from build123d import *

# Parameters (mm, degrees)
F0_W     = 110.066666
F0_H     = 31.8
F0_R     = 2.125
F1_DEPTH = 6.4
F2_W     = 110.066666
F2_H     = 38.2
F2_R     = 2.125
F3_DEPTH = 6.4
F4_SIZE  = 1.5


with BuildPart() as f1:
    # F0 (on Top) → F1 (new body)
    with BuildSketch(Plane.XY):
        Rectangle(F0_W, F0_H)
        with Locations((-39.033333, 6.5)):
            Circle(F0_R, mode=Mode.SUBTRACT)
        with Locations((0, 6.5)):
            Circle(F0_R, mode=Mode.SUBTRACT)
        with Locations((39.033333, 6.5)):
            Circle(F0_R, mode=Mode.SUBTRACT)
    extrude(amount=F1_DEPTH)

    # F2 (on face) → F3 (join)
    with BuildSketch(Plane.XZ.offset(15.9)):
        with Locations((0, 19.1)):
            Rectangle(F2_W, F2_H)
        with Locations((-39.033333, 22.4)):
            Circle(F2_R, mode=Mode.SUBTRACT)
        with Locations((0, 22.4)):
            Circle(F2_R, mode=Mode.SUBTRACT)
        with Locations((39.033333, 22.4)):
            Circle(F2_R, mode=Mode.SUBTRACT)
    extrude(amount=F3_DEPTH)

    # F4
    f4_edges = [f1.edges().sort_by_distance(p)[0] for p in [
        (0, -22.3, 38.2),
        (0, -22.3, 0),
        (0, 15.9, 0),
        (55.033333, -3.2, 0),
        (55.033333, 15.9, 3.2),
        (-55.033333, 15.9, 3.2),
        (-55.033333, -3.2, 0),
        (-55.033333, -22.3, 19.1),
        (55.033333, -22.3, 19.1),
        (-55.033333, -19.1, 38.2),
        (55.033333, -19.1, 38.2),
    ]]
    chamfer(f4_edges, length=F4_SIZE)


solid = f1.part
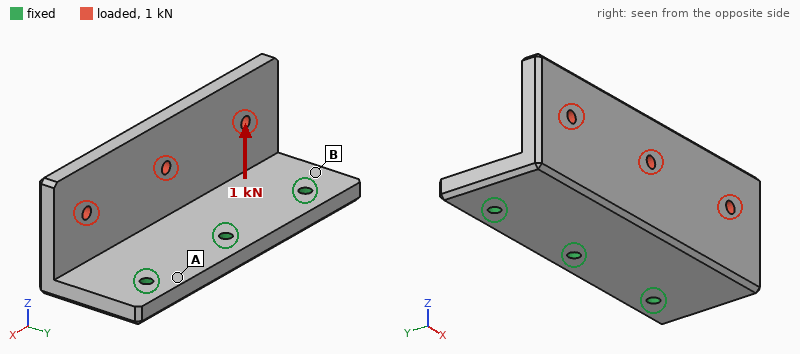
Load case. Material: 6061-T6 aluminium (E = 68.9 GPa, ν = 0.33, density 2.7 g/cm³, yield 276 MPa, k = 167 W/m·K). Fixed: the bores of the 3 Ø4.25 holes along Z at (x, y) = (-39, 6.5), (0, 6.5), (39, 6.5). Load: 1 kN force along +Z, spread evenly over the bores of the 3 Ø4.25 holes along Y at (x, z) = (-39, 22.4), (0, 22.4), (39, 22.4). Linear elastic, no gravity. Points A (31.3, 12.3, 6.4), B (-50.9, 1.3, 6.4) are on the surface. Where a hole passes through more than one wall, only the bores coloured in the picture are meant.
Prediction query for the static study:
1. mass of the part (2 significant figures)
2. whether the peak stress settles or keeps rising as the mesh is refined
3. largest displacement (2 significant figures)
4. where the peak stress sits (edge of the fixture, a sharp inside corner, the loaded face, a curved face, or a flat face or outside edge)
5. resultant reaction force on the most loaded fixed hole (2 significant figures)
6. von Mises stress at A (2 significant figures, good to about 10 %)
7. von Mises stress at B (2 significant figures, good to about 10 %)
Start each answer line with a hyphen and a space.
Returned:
- 130 g
- keeps rising
- 0.10 mm
- edge of the fixture
- 350 N
- 9.4 MPa
- 20 MPa
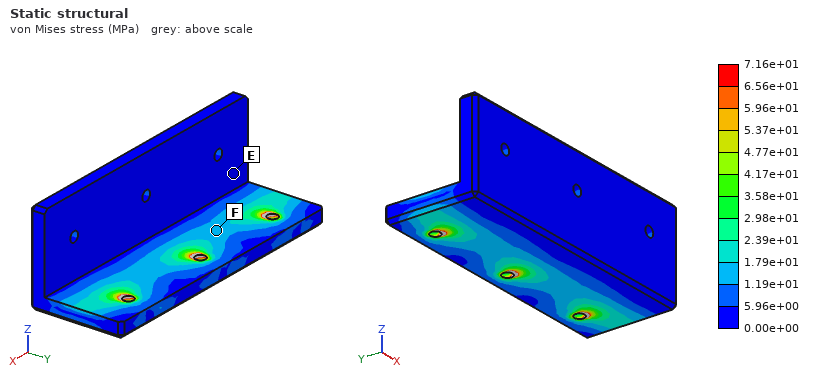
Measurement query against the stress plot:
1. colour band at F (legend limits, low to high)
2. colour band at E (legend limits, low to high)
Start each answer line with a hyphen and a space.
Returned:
- 1.19e+01 to 1.79e+01 MPa
- 0.00e+00 to 5.96e+00 MPa
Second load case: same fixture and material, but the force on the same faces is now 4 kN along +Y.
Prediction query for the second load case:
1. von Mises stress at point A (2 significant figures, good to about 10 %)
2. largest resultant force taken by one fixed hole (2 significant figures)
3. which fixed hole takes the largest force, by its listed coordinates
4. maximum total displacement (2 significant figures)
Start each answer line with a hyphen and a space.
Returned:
- 34 MPa
- 1.5 kN
- (0, 6.5)
- 0.58 mm
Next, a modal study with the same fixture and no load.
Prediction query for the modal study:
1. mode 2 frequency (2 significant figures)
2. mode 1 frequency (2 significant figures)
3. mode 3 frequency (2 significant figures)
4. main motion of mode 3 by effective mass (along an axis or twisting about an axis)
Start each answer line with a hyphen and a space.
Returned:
- 2700 Hz
- 1800 Hz
- 4900 Hz
- along Z
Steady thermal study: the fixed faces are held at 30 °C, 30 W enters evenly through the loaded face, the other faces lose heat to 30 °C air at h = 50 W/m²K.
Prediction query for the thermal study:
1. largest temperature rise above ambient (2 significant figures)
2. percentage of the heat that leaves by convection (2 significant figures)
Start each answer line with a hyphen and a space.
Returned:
- 13 K
- 18 %
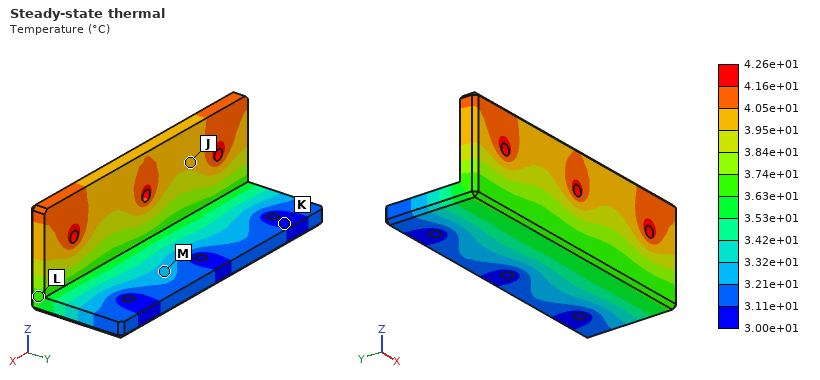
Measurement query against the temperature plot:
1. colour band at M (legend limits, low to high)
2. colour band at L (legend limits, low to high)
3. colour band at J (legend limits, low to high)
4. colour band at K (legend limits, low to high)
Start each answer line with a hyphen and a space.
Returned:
- 3.21e+01 to 3.32e+01 °C
- 3.63e+01 to 3.74e+01 °C
- 3.95e+01 to 4.05e+01 °C
- 3.00e+01 to 3.11e+01 °C
